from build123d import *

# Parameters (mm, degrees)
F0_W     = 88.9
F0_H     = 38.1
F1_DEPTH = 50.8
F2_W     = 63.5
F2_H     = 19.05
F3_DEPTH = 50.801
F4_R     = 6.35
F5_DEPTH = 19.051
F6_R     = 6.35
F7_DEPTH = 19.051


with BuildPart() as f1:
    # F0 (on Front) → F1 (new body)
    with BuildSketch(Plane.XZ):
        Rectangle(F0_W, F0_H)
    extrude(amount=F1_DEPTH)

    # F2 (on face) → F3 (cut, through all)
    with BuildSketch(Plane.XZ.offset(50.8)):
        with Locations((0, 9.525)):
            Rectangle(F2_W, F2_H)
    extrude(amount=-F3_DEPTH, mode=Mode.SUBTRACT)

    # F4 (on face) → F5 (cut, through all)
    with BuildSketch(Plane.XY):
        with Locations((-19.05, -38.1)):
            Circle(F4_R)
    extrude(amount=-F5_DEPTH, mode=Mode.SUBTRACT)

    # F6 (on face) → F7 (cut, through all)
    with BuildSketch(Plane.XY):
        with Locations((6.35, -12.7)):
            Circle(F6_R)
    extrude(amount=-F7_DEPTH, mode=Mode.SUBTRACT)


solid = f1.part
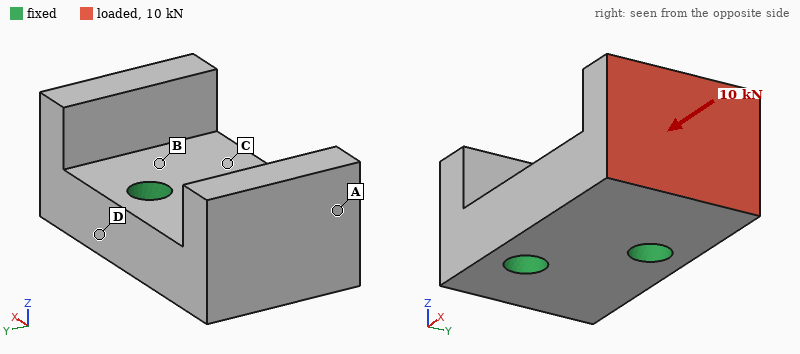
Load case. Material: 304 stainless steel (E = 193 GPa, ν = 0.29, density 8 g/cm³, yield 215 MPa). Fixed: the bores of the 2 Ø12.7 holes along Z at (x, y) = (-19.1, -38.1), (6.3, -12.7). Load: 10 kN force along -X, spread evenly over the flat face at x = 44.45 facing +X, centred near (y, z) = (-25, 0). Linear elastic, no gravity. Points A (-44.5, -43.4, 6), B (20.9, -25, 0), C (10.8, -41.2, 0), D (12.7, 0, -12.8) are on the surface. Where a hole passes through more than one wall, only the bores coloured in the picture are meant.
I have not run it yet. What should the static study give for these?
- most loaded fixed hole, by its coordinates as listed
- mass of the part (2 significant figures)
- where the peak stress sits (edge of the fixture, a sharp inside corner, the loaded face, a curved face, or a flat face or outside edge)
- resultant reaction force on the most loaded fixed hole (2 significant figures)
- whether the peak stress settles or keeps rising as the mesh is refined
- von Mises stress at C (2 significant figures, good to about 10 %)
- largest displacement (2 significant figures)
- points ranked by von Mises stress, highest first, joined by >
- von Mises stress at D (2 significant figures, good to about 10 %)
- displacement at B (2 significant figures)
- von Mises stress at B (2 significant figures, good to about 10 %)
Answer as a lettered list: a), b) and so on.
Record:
a) (6.3, -12.7)
b) 850 g
c) edge of the fixture
d) 6.1 kN
e) keeps rising
f) 29 MPa
g) 29 µm
h) B > C > D > A
i) 14 MPa
j) 4.5 µm
k) 38 MPa
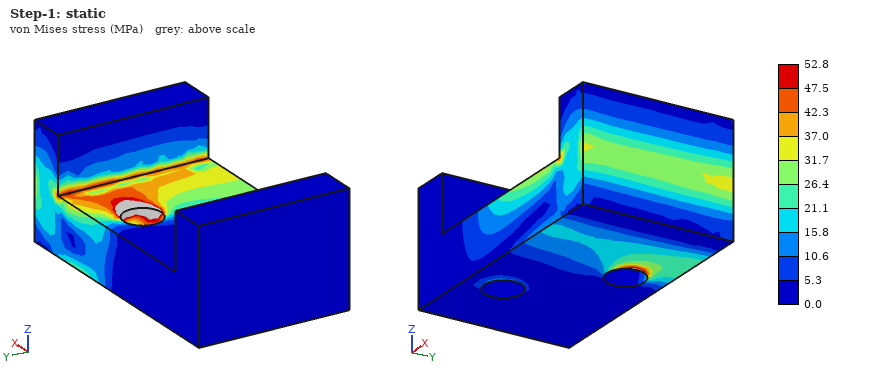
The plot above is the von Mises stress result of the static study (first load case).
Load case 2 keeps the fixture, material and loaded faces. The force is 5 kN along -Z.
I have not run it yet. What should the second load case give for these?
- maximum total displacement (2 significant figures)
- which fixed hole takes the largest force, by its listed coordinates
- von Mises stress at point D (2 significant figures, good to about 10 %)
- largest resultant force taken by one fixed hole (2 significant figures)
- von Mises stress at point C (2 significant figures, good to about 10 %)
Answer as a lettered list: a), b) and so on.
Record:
a) 36 µm
b) (6.3, -12.7)
c) 21 MPa
d) 5.5 kN
e) 30 MPa
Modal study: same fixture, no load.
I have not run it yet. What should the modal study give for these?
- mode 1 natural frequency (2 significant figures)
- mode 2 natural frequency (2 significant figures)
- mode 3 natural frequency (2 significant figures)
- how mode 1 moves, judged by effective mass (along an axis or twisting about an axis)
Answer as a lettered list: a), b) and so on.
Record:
a) 5300 Hz
b) 7600 Hz
c) 7800 Hz
d) along Z
